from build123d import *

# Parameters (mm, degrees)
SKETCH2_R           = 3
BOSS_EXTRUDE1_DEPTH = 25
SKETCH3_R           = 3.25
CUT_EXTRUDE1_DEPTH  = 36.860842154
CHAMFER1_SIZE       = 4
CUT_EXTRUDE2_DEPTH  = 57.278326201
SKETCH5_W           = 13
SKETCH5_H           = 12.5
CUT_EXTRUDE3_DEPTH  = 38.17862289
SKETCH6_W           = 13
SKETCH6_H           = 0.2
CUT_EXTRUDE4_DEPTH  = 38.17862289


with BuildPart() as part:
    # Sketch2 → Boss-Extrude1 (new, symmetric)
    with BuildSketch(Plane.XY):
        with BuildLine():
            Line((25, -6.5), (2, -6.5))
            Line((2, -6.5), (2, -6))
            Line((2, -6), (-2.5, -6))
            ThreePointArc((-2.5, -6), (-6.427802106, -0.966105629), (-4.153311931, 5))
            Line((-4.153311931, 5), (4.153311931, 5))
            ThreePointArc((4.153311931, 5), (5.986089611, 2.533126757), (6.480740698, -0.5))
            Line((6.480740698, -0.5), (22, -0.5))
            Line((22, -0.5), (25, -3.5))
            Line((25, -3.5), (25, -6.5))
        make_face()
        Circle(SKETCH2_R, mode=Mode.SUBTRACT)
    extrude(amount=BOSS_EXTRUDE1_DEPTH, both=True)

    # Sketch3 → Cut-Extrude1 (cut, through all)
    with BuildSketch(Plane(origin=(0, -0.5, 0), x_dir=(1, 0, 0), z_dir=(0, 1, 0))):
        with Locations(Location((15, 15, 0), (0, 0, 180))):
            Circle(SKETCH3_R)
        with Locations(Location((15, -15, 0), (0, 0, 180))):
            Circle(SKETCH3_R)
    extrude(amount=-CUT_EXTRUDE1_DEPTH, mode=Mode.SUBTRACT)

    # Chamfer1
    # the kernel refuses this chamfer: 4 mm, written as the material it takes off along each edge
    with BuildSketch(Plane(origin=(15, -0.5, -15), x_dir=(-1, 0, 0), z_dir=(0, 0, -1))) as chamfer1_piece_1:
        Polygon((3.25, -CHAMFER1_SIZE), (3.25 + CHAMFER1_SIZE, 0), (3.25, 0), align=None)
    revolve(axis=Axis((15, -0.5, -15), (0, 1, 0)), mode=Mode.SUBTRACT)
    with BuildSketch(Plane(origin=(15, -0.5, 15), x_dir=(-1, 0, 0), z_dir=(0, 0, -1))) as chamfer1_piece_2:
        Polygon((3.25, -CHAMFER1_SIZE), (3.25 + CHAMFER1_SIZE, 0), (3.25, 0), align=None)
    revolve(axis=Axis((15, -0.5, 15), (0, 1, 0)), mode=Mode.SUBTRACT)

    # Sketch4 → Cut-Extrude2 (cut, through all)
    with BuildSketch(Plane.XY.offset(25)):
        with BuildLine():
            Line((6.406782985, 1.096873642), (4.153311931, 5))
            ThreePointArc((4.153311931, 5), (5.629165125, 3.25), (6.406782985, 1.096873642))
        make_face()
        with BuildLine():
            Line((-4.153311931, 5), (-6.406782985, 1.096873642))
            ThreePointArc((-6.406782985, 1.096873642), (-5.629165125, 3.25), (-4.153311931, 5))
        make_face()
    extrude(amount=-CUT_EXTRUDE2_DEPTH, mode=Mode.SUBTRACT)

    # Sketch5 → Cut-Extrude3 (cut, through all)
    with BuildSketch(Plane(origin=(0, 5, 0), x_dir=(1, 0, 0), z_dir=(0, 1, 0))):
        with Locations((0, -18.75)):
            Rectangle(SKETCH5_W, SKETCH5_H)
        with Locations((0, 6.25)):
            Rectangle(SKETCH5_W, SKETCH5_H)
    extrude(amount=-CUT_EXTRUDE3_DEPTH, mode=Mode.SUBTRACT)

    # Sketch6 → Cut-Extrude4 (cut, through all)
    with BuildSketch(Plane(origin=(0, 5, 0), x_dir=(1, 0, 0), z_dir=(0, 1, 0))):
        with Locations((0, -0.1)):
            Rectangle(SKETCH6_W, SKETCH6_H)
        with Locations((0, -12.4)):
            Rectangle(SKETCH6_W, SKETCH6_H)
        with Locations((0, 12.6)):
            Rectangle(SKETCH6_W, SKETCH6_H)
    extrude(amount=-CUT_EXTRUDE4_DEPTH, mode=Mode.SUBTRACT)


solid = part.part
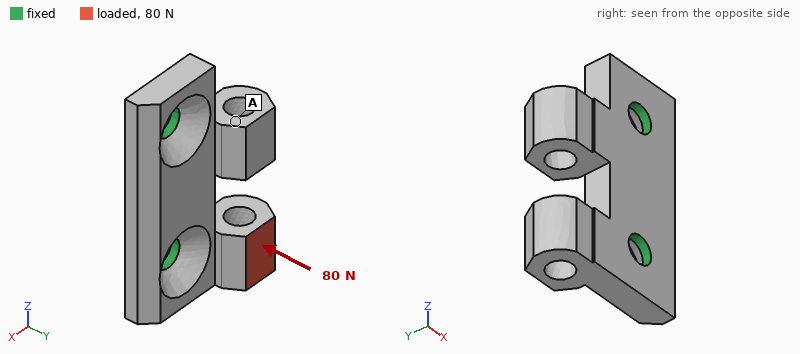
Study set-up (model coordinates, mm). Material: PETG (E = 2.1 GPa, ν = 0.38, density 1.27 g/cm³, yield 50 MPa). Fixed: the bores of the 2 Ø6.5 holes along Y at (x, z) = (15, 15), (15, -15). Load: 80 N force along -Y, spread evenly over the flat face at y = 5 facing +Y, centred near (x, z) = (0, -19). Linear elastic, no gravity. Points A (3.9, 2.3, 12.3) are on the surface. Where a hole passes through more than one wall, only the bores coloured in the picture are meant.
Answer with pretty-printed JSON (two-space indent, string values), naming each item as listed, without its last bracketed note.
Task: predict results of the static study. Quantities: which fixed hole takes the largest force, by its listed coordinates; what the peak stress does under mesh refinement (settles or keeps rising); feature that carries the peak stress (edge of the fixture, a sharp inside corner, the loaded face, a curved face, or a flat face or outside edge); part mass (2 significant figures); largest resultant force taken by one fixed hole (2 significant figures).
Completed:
{
  "which fixed hole takes the largest force, by its listed coordinates": "(15, -15)",
  "what the peak stress does under mesh refinement": "keeps rising",
  "feature that carries the peak stress": "a sharp inside corner",
  "part mass": "8.8 g",
  "largest resultant force taken by one fixed hole": "89 N"
}
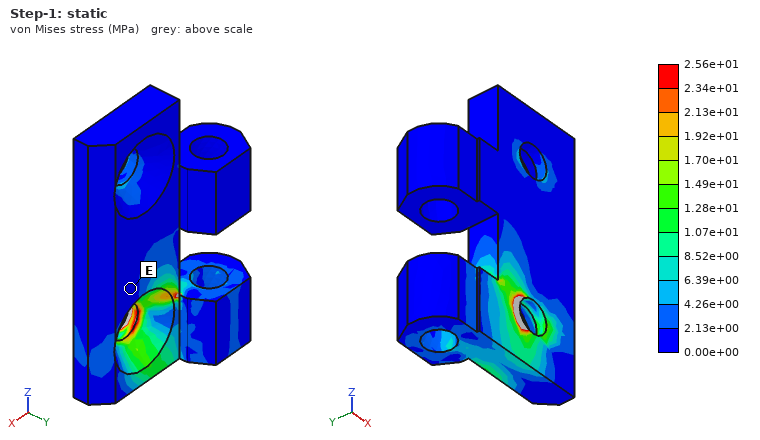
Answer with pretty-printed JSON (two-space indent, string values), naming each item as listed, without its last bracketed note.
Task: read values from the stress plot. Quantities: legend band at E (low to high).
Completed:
{
  "legend band at E": "0.00e+00 to 2.13e+00 MPa"
}
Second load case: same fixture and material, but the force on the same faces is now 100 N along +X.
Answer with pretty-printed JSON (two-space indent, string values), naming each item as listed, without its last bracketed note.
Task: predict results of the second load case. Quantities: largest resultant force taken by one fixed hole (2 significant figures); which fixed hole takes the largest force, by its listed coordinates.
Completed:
{
  "largest resultant force taken by one fixed hole": "97 N",
  "which fixed hole takes the largest force, by its listed coordinates": "(15, -15)"
}
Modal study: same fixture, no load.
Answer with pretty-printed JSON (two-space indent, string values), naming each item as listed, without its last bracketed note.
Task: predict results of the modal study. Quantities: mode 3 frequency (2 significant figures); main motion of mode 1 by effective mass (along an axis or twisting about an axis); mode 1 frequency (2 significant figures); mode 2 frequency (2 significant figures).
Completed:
{
  "mode 3 frequency": "3600 Hz",
  "main motion of mode 1 by effective mass": "along Y",
  "mode 1 frequency": "1600 Hz",
  "mode 2 frequency": "1900 Hz"
}
